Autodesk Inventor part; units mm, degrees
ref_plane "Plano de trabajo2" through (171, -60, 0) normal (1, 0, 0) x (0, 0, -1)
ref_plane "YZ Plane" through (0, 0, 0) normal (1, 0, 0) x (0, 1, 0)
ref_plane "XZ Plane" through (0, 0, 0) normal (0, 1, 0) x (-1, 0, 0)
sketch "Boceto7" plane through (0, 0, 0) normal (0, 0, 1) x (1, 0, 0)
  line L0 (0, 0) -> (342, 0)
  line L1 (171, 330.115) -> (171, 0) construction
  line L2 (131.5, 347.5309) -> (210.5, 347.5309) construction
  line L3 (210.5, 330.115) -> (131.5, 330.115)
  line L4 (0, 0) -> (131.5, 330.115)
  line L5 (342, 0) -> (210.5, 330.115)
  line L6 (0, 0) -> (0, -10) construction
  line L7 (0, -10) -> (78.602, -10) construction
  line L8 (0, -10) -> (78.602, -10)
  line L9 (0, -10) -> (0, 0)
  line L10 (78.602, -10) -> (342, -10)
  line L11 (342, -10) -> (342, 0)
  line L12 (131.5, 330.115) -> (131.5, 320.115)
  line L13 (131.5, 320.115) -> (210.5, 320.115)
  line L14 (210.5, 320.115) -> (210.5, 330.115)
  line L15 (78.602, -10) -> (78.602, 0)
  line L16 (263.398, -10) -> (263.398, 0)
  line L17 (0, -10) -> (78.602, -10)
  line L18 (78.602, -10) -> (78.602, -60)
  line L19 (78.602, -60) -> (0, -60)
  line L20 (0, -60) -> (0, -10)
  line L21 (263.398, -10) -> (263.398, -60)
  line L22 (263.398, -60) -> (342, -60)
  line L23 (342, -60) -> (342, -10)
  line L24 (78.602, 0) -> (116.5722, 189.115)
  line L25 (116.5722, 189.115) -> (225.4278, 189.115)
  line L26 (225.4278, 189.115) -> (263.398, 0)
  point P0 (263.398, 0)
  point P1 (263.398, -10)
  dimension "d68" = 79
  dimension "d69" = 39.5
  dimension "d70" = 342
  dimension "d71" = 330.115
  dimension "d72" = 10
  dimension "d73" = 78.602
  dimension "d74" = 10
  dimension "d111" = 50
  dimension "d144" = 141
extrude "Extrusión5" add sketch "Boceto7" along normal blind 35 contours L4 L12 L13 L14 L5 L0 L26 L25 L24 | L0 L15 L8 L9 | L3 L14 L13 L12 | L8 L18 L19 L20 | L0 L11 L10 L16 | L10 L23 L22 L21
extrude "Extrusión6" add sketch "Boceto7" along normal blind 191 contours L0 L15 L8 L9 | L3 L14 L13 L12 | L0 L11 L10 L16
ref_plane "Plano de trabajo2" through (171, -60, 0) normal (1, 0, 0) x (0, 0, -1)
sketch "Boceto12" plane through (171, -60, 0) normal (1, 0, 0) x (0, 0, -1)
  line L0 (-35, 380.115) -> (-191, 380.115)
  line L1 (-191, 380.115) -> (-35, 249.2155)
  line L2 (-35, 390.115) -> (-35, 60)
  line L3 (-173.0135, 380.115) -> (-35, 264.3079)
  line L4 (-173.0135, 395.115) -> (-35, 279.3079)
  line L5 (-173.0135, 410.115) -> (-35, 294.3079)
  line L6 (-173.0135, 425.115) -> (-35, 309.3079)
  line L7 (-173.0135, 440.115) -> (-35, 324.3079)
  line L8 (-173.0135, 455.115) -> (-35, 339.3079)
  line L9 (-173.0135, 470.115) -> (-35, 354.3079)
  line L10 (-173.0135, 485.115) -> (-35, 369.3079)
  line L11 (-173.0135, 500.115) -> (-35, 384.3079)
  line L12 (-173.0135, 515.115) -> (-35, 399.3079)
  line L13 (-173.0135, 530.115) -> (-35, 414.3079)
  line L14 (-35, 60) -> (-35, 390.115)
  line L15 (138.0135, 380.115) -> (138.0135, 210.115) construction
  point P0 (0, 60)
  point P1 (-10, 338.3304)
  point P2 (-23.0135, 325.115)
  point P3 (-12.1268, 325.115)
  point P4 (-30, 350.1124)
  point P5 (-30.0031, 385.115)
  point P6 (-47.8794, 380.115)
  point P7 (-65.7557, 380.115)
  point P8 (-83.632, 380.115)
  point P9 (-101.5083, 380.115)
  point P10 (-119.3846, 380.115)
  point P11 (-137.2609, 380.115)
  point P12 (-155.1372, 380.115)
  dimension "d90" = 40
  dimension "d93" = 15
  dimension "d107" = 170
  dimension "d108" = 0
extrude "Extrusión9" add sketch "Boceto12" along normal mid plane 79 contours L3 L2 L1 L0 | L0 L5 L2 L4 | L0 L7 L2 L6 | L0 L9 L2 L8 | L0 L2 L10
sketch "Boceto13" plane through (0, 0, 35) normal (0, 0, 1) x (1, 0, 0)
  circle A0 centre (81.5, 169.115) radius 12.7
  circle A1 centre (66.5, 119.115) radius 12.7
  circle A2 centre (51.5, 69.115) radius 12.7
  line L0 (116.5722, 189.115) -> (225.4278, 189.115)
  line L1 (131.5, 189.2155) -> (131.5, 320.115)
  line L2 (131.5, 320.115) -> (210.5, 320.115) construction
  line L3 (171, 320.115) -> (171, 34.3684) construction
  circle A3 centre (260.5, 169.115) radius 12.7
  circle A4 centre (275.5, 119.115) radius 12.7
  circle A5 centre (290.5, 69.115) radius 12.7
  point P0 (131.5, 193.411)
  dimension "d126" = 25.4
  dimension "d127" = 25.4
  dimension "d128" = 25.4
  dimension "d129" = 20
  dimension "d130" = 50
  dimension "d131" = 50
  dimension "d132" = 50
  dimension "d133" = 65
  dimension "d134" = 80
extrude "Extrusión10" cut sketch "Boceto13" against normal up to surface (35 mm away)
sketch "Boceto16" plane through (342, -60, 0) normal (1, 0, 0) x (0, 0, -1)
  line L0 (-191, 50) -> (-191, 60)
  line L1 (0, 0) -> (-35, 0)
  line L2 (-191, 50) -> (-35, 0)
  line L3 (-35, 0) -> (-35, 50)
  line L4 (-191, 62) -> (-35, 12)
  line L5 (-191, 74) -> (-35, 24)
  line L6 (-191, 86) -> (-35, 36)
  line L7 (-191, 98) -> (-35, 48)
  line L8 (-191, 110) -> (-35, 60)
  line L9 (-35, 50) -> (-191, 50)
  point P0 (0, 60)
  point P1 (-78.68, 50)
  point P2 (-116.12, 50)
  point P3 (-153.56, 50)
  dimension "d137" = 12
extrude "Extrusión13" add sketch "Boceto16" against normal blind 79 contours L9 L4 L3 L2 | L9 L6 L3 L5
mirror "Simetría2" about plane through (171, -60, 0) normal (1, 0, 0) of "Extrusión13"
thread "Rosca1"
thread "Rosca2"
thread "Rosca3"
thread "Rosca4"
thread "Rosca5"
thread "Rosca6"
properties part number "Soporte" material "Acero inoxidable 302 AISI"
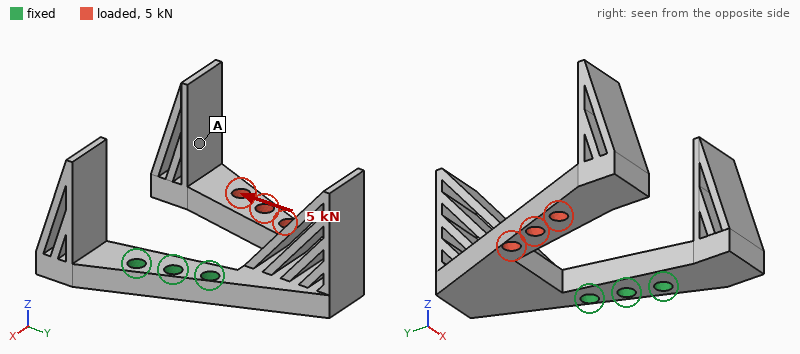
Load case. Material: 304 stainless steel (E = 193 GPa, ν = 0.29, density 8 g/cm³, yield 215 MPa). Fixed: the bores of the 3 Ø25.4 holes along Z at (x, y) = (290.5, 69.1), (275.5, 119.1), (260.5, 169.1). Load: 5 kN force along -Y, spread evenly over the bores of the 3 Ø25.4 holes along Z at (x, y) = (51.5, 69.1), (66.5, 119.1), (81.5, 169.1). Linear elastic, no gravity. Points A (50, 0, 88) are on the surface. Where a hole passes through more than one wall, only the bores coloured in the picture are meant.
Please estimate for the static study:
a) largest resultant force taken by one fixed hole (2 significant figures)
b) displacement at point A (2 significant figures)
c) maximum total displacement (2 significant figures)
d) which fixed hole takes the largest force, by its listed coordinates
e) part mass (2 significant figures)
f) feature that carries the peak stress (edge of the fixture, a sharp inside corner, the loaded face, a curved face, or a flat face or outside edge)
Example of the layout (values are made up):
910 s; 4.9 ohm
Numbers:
6.9 kN; 0.48 mm; 0.64 mm; (275.5, 119.1); 23 kg; the loaded face
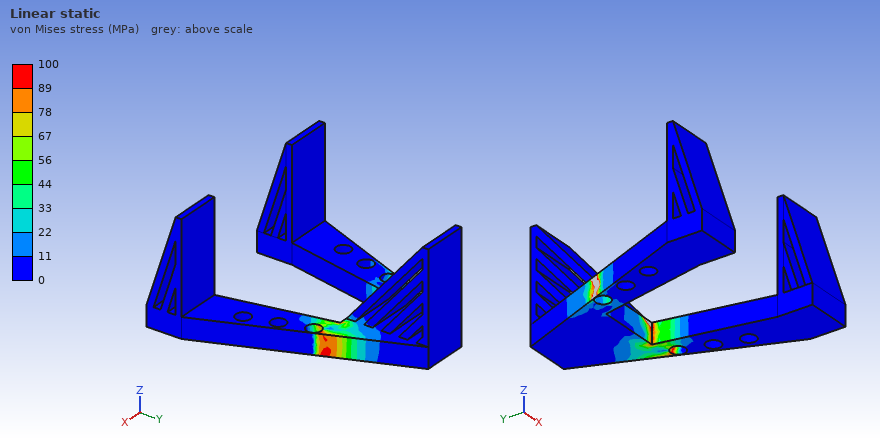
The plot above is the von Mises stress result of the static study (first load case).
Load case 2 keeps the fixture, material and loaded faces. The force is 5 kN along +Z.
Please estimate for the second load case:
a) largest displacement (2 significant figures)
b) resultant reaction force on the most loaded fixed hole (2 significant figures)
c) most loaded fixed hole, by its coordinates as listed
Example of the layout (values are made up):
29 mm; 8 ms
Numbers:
1.4 mm; 4.9 kN; (260.5, 169.1)
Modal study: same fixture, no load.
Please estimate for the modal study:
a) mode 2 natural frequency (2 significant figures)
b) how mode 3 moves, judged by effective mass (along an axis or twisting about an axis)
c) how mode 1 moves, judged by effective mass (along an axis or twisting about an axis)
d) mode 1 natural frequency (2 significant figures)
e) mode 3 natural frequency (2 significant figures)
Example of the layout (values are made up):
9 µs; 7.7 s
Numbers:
120 Hz; along Z; along Z; 95 Hz; 250 Hz
